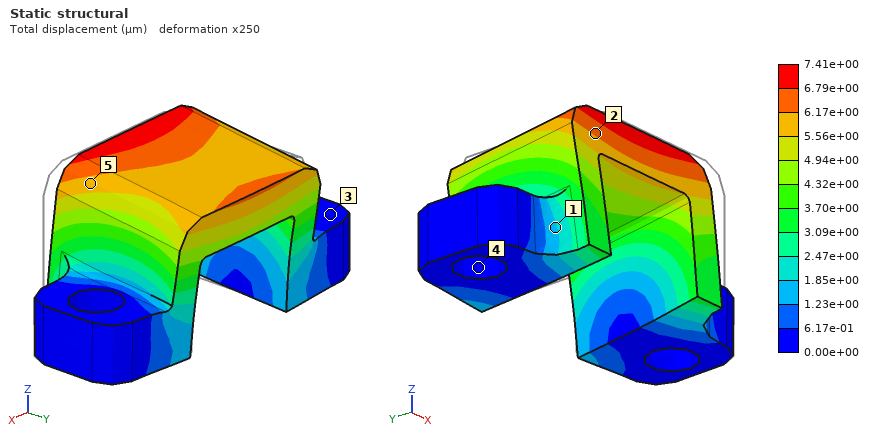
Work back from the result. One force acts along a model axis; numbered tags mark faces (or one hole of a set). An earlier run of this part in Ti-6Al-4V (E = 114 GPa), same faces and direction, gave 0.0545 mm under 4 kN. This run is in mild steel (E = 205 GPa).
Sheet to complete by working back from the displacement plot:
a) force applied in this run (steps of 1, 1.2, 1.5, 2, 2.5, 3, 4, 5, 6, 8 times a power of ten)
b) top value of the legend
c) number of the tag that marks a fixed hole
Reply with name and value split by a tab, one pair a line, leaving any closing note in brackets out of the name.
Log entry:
force applied in this run	1 kN
top value of the legend	7.41e+00 µm
number of the tag that marks a fixed hole	4
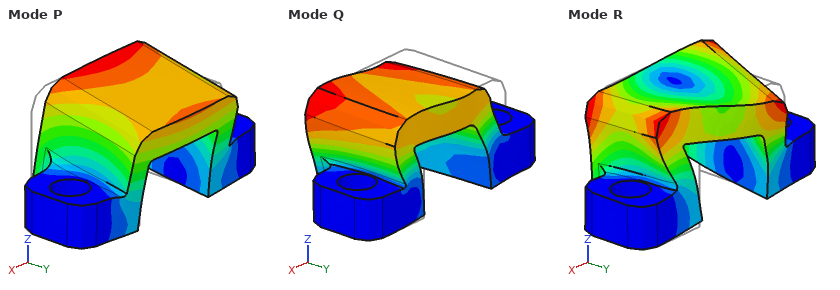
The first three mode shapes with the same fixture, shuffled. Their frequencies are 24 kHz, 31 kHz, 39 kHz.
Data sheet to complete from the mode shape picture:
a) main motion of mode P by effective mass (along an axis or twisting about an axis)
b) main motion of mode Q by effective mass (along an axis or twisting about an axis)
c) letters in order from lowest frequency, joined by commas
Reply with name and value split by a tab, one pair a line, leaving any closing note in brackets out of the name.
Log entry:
main motion of mode P by effective mass	along Y
main motion of mode Q by effective mass	along X
letters in order from lowest frequency, joined by commas	P, Q, R
